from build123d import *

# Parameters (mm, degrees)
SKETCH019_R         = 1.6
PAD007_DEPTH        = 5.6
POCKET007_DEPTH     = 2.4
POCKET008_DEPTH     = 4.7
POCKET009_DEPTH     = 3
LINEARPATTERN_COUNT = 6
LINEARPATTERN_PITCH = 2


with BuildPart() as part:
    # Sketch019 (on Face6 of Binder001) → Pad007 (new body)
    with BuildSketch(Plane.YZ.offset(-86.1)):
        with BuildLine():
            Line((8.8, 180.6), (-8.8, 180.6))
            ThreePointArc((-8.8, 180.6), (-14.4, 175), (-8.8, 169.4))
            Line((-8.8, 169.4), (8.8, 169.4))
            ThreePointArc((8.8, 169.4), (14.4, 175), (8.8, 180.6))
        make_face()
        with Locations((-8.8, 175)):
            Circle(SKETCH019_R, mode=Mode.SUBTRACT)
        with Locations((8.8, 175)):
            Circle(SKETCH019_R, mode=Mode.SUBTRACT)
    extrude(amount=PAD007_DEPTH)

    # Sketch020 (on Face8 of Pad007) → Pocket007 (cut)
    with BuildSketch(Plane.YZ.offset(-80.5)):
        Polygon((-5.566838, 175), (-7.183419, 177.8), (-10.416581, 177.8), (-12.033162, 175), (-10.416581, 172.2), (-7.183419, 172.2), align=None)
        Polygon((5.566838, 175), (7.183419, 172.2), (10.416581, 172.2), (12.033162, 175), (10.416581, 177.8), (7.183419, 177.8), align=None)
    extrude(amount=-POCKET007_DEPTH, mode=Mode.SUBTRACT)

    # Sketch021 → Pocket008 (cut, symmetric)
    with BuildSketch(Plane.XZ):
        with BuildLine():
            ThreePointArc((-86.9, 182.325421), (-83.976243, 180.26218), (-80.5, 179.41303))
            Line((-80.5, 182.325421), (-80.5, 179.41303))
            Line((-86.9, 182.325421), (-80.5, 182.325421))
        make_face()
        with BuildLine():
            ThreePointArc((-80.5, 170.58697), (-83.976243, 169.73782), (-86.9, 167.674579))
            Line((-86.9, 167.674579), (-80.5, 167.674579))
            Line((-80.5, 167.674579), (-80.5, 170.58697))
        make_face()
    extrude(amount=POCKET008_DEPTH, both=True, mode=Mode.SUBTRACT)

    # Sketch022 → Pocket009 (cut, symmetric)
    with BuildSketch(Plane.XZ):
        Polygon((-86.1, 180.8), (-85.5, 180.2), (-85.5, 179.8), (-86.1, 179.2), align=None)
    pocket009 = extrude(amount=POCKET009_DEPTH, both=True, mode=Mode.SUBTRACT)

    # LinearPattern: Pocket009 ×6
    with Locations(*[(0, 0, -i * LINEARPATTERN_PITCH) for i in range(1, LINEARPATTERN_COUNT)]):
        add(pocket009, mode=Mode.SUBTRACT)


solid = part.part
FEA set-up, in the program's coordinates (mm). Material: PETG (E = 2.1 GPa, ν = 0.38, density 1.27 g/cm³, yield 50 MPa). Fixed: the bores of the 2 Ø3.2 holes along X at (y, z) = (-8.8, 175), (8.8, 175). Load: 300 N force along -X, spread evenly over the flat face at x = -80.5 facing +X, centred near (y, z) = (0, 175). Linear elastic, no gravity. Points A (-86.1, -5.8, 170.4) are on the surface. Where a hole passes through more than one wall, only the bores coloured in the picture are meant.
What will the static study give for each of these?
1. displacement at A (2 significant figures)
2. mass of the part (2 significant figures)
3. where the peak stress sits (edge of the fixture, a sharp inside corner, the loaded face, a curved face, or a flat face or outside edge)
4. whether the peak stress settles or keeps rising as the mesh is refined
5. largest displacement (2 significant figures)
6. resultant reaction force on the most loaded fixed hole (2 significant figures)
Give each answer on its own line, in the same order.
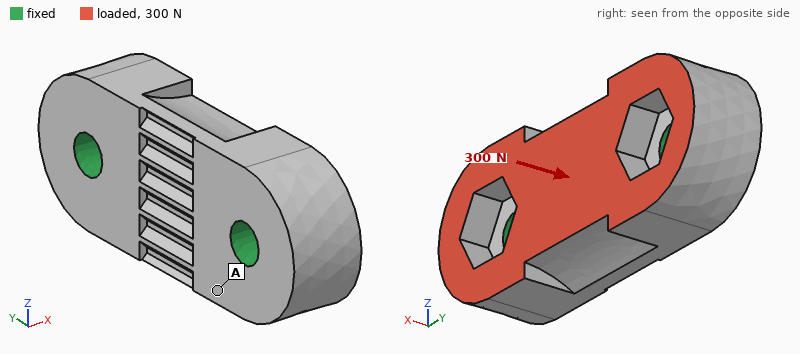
21 µm
1.8 g
edge of the fixture
keeps rising
34 µm
150 N
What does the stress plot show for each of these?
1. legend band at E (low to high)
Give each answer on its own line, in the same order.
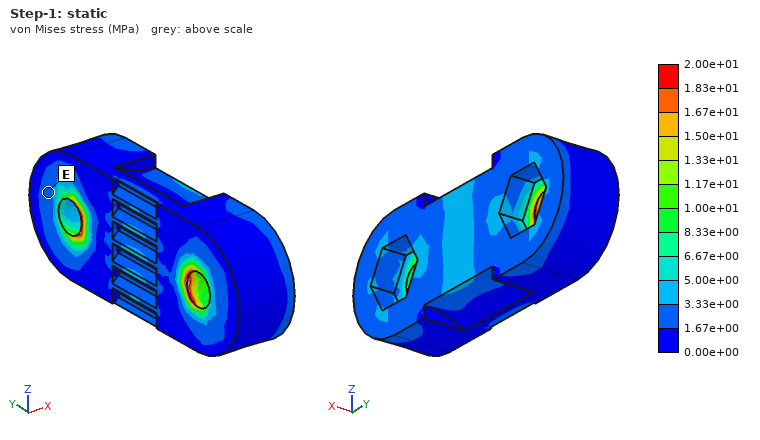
1.67e+00 to 3.33e+00 MPa
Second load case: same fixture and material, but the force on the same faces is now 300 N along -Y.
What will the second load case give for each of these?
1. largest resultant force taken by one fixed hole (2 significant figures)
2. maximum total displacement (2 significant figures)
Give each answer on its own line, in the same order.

160 N
39 µm
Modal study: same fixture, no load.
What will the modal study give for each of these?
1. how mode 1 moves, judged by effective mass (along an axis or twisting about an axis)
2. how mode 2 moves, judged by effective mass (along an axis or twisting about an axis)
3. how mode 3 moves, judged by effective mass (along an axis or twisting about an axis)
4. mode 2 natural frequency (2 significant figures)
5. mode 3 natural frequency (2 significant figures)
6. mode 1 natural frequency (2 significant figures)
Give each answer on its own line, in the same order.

along Z
along X
along Z
13 kHz
16 kHz
11 kHz
